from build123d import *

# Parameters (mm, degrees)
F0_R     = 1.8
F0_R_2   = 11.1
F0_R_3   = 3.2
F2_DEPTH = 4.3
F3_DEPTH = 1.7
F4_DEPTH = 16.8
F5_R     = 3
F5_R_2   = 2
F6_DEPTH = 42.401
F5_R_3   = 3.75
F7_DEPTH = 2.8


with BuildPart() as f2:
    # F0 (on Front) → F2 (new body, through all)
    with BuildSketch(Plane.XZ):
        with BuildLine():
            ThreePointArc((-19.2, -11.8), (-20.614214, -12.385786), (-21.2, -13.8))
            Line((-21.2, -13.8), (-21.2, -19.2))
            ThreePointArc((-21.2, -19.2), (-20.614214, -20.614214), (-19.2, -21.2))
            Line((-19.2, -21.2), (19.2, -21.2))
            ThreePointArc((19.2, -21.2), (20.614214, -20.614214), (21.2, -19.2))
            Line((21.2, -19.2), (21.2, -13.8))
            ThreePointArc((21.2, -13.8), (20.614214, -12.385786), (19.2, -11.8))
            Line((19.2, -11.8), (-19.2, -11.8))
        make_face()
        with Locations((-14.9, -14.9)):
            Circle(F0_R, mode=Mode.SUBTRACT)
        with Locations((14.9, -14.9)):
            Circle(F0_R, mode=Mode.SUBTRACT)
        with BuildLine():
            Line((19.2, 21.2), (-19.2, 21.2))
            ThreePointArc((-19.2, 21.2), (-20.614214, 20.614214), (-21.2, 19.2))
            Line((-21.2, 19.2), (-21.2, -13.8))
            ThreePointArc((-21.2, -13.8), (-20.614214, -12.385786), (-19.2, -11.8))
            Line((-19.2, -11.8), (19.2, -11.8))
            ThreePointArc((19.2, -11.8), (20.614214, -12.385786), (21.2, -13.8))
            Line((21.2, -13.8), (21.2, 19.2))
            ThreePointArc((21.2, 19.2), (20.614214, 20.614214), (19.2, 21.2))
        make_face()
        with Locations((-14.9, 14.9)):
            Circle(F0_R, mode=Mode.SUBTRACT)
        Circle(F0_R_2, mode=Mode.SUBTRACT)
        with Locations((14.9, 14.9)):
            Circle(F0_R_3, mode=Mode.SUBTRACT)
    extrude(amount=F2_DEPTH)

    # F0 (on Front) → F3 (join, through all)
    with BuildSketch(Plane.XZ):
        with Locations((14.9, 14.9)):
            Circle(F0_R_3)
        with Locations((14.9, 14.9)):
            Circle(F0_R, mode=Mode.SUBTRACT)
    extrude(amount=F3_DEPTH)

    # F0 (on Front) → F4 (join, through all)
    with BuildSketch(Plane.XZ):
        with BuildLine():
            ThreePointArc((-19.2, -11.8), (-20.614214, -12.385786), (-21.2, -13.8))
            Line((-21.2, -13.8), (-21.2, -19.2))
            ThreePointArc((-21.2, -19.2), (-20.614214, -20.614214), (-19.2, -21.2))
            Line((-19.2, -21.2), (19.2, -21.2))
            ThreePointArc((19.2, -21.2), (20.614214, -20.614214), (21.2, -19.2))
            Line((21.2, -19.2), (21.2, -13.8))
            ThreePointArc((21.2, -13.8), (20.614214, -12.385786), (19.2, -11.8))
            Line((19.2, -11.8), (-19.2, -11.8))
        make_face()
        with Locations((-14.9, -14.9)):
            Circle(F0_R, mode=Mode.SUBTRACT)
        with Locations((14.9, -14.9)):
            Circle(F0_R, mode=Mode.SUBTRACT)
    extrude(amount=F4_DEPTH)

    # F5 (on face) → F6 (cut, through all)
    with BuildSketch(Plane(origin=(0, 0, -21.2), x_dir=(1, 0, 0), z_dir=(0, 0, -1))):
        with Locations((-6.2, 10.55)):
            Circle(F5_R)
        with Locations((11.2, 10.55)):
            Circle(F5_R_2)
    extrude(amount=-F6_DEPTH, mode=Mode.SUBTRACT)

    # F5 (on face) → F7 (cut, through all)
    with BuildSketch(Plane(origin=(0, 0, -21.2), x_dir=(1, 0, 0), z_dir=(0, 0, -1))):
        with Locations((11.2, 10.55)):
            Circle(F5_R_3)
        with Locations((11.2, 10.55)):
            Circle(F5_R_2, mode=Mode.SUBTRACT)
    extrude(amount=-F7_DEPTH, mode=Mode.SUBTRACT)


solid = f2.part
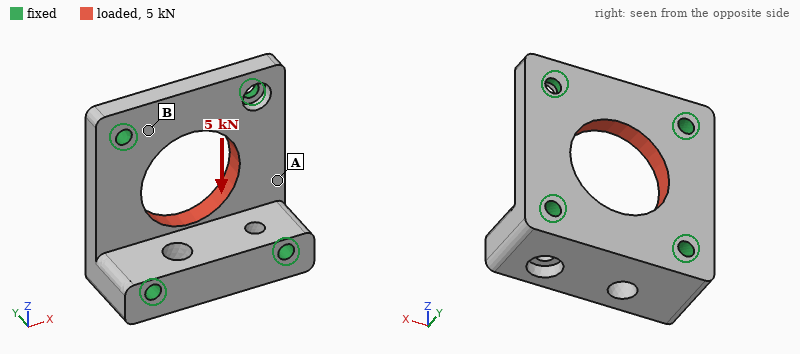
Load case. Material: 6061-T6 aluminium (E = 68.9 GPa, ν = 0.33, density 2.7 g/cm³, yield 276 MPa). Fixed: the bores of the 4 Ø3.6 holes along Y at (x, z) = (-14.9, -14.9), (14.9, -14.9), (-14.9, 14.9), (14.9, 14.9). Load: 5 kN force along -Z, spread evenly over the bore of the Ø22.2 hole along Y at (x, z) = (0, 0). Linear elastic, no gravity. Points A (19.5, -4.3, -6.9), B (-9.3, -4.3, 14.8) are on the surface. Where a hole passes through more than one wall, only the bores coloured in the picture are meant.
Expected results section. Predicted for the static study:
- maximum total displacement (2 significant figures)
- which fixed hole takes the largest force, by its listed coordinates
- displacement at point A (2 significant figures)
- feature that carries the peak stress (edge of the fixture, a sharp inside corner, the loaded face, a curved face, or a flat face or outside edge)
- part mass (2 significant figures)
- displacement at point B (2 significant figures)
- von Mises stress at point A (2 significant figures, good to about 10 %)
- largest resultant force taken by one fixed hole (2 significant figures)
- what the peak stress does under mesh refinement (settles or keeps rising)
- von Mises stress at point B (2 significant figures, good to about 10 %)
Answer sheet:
13 µm
(14.9, -14.9)
2.1 µm
edge of the fixture
27 g
4.8 µm
11 MPa
1.5 kN
keeps rising
28 MPa
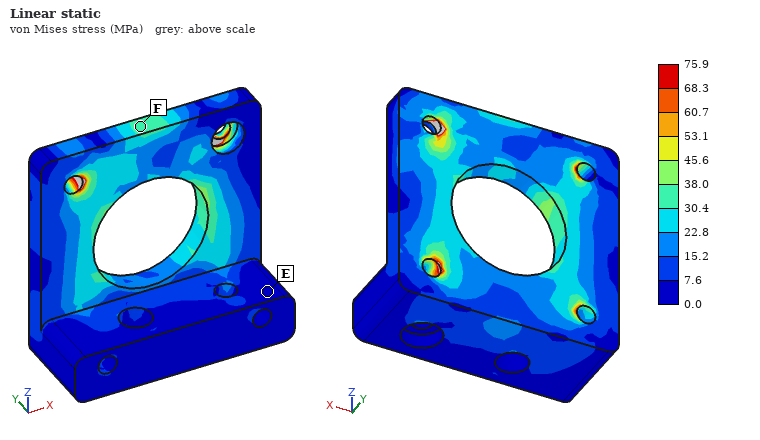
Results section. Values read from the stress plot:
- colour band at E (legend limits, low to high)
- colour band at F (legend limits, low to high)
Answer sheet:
0.0 to 7.6 MPa
30.4 to 38.0 MPa
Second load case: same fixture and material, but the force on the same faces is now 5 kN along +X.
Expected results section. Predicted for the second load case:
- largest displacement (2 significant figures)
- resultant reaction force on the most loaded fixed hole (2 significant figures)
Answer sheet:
12 µm
1.4 kN
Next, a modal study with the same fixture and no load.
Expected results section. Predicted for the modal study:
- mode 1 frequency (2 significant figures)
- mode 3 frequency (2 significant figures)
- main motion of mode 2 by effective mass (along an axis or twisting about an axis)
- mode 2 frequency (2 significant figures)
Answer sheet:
20 kHz
26 kHz
along Y
22 kHz
